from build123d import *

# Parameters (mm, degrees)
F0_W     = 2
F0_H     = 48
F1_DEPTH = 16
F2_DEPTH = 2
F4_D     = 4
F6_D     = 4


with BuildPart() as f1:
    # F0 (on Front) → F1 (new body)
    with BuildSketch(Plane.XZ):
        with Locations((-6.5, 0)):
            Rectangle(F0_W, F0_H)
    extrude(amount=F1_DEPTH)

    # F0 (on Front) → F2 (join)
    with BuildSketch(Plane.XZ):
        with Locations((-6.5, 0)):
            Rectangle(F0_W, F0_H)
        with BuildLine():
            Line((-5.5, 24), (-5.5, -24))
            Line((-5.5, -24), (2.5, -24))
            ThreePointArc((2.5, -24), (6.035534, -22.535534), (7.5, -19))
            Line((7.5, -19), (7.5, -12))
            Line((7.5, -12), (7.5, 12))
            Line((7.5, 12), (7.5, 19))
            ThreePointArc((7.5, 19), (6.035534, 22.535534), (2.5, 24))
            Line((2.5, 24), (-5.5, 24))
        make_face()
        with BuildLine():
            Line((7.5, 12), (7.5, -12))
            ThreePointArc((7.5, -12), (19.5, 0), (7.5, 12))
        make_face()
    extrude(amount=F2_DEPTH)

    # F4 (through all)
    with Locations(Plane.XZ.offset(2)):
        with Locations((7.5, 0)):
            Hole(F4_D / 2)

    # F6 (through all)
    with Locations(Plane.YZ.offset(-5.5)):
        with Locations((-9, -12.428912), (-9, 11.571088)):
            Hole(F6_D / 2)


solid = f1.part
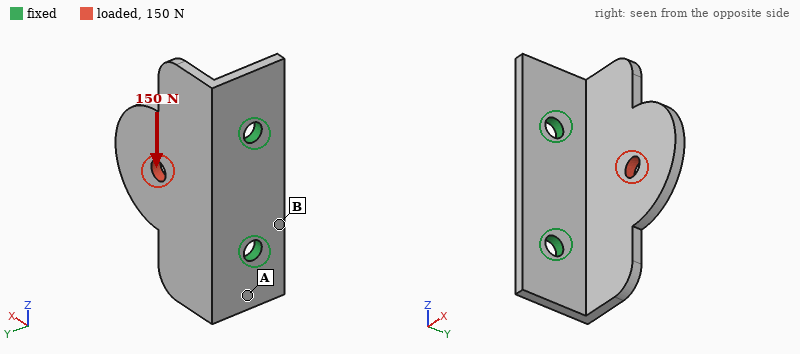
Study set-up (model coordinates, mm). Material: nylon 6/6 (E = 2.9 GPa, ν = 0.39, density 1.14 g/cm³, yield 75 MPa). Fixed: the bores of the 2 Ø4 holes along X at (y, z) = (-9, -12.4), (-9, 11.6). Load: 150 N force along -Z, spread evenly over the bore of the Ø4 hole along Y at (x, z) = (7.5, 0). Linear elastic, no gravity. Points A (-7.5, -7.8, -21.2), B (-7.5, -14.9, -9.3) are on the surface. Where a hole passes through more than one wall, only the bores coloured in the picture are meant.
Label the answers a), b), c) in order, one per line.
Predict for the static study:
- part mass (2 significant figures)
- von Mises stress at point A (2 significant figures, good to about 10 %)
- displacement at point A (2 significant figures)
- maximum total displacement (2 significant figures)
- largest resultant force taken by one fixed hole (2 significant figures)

a) 3.6 g
b) 10 MPa
c) 0.11 mm
d) 0.62 mm
e) 120 N
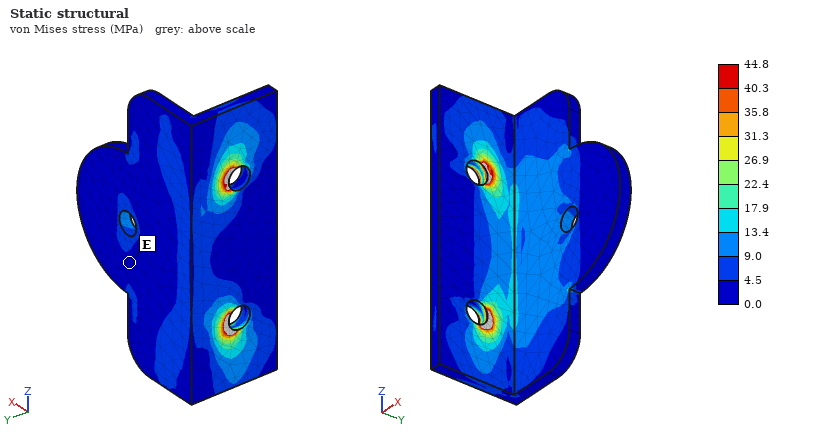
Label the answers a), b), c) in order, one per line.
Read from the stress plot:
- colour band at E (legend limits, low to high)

a) 0.0 to 4.5 MPa
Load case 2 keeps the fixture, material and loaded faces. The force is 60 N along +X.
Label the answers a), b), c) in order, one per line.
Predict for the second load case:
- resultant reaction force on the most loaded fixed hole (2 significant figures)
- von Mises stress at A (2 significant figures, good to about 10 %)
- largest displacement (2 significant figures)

a) 31 N
b) 4.2 MPa
c) 0.52 mm
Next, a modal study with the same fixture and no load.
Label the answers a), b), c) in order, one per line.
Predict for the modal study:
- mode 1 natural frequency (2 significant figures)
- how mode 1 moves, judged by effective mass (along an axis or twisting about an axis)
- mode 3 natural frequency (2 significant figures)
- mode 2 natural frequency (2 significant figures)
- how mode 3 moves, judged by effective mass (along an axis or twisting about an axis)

a) 800 Hz
b) along Y
c) 2600 Hz
d) 1700 Hz
e) along X
